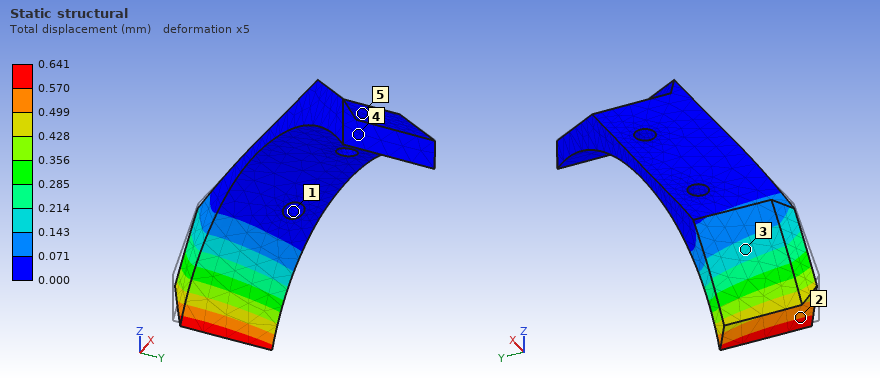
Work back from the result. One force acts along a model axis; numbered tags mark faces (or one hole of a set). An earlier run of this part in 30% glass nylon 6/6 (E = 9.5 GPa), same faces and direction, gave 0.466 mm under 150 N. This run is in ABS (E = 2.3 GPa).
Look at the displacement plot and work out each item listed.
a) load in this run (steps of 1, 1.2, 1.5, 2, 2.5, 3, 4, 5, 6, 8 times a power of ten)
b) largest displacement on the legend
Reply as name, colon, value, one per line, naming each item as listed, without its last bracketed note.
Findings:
load in this run: 50 N
largest displacement on the legend: 0.641 mm
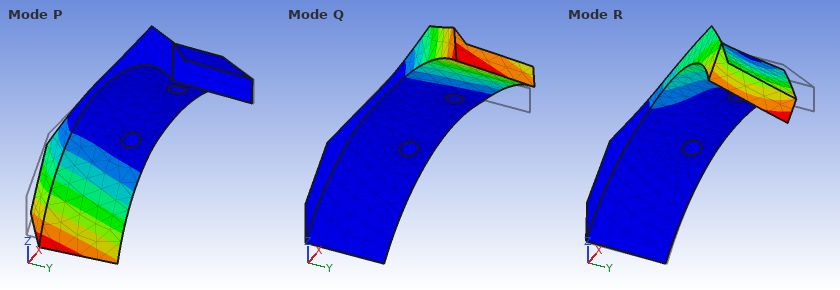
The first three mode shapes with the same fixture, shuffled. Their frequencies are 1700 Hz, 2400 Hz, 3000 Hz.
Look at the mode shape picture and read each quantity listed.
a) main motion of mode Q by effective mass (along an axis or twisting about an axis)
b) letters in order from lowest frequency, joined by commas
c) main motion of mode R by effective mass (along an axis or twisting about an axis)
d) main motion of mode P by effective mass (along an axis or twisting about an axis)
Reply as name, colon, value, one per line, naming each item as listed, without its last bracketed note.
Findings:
main motion of mode Q by effective mass: along Z
letters in order from lowest frequency, joined by commas: Q, P, R
main motion of mode R by effective mass: along Y
main motion of mode P by effective mass: along Z
